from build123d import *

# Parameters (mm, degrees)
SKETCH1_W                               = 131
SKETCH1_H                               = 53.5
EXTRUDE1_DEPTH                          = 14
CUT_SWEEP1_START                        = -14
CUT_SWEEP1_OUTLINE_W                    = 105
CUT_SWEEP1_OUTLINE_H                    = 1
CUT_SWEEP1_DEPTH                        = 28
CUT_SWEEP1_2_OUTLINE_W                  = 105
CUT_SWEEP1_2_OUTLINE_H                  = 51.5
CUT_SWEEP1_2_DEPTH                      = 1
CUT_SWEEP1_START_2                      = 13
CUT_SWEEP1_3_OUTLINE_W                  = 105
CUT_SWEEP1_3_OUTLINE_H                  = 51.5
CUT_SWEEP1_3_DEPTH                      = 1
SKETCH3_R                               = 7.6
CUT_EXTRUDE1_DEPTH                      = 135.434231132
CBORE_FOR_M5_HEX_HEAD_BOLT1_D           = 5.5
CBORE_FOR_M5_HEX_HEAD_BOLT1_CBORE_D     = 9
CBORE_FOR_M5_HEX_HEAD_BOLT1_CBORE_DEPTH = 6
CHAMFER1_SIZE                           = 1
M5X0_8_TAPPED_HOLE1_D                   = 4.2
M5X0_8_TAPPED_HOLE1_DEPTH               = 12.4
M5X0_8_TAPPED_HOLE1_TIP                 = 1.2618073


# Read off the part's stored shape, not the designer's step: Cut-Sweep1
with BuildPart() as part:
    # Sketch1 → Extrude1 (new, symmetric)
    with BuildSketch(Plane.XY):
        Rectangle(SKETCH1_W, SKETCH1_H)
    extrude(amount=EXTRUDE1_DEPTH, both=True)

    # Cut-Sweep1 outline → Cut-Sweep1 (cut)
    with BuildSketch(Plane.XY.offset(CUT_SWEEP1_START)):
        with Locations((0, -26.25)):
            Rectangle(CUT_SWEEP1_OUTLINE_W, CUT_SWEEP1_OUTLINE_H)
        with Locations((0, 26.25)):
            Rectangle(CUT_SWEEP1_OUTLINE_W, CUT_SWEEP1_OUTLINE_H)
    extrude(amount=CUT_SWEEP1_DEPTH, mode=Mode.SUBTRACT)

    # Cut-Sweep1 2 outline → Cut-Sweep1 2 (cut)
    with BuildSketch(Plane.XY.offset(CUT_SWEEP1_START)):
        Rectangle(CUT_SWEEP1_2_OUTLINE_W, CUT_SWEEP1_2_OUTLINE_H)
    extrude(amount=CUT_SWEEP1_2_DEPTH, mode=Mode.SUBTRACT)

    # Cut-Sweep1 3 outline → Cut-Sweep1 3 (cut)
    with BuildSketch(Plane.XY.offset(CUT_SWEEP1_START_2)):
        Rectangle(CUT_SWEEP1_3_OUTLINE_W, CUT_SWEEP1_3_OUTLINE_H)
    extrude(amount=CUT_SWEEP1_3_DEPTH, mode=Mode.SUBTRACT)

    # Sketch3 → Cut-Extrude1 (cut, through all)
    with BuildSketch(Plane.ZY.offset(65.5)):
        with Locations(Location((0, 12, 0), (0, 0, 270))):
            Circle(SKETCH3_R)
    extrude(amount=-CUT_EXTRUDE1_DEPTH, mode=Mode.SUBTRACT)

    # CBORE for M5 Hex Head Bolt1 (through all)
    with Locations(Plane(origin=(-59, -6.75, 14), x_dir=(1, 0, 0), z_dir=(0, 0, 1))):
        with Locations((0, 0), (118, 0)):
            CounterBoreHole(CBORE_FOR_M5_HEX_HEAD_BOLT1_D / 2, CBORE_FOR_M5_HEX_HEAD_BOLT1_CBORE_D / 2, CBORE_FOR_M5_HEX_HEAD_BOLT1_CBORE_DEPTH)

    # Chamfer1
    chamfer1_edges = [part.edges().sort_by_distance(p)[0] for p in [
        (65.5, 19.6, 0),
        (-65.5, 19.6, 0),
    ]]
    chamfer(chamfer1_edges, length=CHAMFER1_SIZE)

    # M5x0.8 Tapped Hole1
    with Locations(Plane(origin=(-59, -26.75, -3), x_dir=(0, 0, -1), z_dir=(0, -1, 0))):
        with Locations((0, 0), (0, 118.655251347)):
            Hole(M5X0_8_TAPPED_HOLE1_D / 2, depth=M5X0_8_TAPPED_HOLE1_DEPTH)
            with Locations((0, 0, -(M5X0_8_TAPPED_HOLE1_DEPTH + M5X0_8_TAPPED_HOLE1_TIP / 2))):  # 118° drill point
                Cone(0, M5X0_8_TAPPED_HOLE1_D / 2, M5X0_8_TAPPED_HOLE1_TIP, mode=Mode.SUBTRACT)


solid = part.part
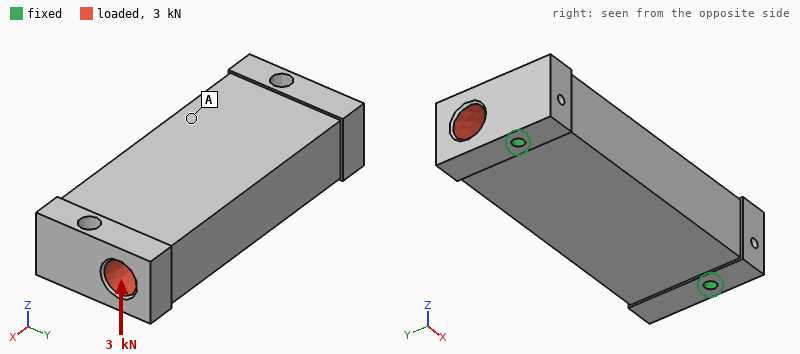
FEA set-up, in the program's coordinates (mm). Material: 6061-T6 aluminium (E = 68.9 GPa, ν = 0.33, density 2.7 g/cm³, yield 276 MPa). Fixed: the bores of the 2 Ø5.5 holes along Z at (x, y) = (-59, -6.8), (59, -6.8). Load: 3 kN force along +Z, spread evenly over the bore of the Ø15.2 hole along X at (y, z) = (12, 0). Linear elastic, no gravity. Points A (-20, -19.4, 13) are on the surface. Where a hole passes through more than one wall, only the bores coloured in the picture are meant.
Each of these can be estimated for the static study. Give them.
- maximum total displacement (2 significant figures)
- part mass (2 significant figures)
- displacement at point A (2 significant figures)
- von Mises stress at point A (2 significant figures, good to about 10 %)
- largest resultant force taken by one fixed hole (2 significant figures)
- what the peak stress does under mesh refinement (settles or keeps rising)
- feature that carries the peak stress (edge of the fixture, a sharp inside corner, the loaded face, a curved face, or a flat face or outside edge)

19 µm
410 g
4.9 µm
3.2 MPa
1.5 kN
keeps rising
edge of the fixture
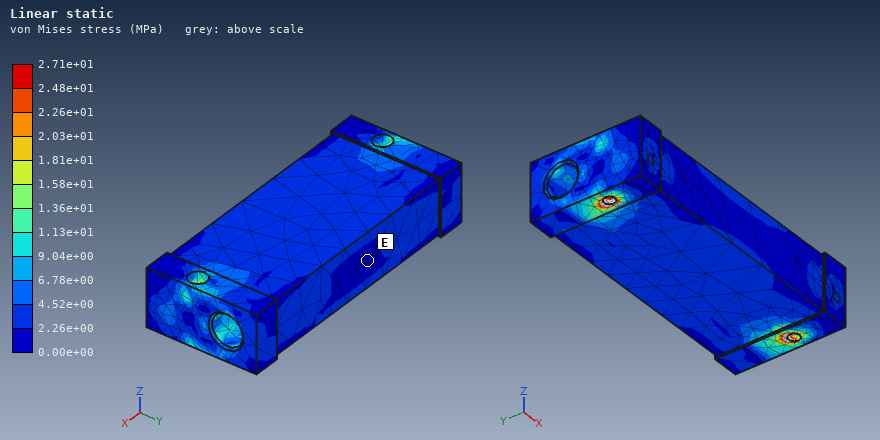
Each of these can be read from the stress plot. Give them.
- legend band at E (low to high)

0.00e+00 to 2.26e+00 MPa
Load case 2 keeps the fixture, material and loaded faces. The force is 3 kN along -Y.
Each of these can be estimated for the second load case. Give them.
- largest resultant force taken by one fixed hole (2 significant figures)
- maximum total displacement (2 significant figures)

1.5 kN
5.3 µm
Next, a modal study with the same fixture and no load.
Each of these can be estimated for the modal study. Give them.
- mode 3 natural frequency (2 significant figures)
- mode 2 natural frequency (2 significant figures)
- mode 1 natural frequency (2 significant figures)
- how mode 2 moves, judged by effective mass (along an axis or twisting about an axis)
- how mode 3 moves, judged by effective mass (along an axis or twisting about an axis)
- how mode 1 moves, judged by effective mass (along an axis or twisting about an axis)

7200 Hz
6700 Hz
5200 Hz
along Y
along Y
along Z
